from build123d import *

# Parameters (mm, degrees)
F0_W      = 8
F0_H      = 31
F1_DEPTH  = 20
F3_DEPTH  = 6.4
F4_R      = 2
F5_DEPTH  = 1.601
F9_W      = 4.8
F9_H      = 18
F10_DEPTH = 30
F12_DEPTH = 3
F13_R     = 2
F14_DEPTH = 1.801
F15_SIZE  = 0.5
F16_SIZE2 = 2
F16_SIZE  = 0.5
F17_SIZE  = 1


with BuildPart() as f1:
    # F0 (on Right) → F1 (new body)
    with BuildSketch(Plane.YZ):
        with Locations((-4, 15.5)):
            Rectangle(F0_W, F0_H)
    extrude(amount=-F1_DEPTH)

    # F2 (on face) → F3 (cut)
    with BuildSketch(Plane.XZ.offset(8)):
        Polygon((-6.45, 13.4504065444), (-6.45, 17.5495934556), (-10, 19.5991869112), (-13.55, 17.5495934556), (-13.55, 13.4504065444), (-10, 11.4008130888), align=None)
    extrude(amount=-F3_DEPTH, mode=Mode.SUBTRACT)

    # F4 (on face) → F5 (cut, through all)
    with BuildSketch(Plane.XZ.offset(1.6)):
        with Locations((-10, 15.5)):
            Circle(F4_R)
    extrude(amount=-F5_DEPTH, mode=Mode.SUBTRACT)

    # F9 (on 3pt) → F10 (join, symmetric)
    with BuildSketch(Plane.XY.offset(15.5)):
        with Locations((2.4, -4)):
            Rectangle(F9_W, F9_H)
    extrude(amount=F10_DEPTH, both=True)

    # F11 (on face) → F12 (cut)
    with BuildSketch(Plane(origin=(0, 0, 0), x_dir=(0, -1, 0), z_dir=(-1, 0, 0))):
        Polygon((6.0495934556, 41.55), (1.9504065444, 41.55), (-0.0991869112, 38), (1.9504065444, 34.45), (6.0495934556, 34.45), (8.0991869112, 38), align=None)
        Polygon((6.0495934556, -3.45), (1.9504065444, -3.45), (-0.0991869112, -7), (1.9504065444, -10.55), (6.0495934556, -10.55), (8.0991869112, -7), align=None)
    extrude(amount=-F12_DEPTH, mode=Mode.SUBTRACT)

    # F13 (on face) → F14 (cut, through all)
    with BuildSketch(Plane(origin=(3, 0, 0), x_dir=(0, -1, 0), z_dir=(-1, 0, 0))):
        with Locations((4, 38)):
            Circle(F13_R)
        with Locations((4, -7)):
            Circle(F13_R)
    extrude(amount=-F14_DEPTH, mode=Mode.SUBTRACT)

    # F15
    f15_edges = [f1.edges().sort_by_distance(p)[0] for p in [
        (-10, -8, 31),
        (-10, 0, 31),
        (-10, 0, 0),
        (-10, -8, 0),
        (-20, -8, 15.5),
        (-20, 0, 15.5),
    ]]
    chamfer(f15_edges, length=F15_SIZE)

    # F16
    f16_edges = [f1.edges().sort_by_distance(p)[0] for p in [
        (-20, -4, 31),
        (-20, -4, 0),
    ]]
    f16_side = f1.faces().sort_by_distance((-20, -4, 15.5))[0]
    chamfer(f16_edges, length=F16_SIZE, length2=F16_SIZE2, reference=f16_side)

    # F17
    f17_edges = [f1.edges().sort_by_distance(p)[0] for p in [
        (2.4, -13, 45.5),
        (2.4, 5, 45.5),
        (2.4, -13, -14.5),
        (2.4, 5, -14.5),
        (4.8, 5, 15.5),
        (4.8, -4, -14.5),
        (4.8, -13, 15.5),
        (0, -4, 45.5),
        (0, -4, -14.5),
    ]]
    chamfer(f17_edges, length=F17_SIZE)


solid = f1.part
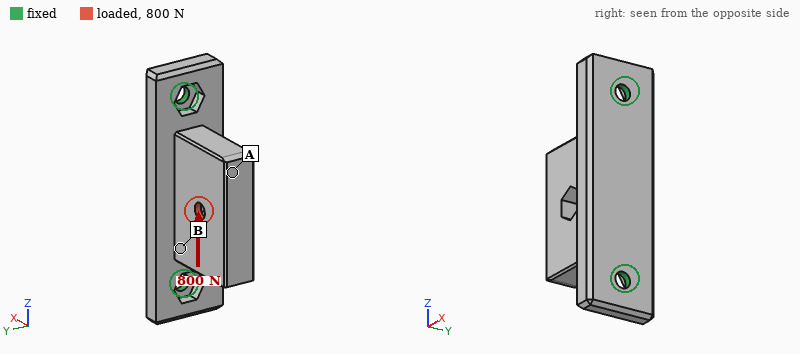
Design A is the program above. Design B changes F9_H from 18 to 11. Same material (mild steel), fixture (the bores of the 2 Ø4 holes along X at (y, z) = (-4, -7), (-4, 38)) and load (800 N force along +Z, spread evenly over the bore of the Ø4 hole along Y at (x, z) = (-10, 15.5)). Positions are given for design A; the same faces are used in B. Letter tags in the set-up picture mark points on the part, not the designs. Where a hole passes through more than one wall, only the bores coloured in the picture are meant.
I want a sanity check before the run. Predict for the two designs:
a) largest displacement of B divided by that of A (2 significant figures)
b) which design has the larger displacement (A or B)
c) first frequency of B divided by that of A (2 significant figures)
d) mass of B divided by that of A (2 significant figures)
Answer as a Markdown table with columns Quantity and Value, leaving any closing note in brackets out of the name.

| Quantity | Value |
|---|---|
| largest displacement of B divided by that of A | 1.1 |
| which design has the larger displacement | B |
| first frequency of B divided by that of A | 0.90 |
| mass of B divided by that of A | 0.79 |
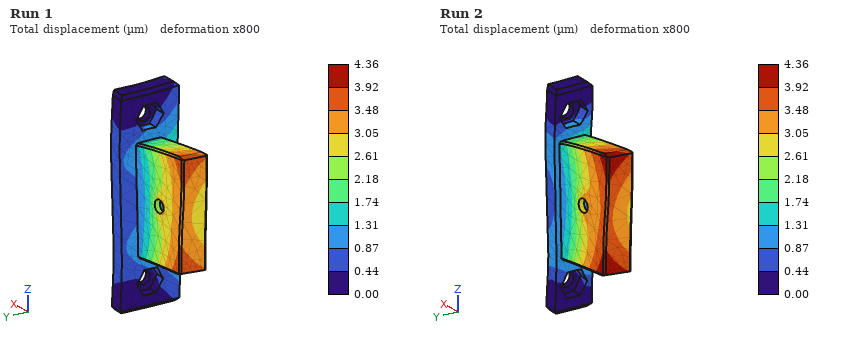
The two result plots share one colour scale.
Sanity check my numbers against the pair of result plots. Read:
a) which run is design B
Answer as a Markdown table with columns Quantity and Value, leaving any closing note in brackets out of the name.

| Quantity | Value |
|---|---|
| which run is design B | Run 2 |
